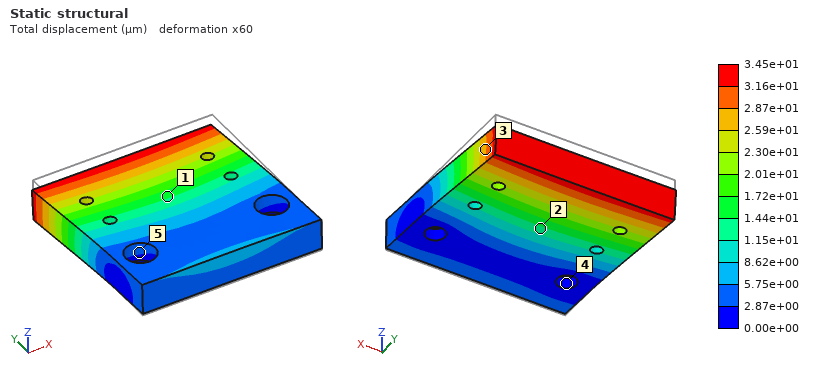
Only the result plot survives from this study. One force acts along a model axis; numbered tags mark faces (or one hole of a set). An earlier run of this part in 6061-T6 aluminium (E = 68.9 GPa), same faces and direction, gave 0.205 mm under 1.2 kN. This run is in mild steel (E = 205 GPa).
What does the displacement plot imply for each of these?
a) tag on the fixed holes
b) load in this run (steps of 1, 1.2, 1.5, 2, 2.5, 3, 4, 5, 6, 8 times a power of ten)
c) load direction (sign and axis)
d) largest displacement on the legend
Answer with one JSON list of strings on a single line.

["4", "600 N", "-Z", "3.45e+01 µm"]
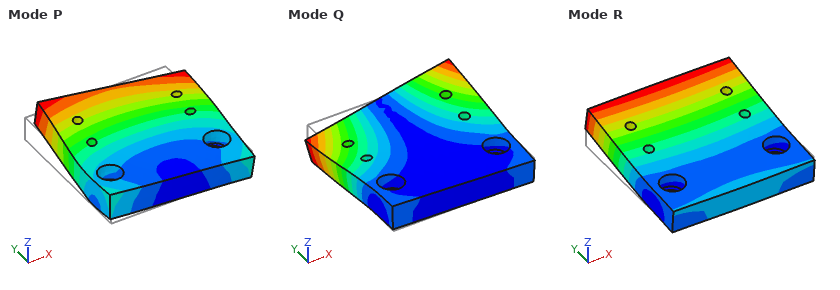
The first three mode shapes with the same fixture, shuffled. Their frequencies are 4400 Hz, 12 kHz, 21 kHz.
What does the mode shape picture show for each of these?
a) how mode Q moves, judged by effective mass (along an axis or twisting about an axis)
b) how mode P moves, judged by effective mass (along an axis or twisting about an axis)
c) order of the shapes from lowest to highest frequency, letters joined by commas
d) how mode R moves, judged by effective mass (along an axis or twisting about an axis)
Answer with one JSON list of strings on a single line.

["twisting about Y", "along X", "R, Q, P", "along Z"]
